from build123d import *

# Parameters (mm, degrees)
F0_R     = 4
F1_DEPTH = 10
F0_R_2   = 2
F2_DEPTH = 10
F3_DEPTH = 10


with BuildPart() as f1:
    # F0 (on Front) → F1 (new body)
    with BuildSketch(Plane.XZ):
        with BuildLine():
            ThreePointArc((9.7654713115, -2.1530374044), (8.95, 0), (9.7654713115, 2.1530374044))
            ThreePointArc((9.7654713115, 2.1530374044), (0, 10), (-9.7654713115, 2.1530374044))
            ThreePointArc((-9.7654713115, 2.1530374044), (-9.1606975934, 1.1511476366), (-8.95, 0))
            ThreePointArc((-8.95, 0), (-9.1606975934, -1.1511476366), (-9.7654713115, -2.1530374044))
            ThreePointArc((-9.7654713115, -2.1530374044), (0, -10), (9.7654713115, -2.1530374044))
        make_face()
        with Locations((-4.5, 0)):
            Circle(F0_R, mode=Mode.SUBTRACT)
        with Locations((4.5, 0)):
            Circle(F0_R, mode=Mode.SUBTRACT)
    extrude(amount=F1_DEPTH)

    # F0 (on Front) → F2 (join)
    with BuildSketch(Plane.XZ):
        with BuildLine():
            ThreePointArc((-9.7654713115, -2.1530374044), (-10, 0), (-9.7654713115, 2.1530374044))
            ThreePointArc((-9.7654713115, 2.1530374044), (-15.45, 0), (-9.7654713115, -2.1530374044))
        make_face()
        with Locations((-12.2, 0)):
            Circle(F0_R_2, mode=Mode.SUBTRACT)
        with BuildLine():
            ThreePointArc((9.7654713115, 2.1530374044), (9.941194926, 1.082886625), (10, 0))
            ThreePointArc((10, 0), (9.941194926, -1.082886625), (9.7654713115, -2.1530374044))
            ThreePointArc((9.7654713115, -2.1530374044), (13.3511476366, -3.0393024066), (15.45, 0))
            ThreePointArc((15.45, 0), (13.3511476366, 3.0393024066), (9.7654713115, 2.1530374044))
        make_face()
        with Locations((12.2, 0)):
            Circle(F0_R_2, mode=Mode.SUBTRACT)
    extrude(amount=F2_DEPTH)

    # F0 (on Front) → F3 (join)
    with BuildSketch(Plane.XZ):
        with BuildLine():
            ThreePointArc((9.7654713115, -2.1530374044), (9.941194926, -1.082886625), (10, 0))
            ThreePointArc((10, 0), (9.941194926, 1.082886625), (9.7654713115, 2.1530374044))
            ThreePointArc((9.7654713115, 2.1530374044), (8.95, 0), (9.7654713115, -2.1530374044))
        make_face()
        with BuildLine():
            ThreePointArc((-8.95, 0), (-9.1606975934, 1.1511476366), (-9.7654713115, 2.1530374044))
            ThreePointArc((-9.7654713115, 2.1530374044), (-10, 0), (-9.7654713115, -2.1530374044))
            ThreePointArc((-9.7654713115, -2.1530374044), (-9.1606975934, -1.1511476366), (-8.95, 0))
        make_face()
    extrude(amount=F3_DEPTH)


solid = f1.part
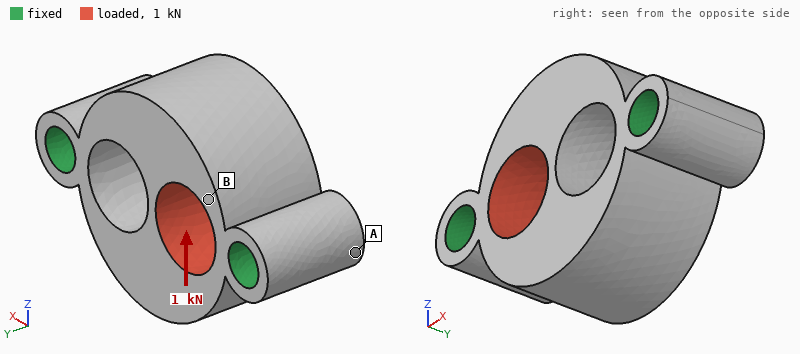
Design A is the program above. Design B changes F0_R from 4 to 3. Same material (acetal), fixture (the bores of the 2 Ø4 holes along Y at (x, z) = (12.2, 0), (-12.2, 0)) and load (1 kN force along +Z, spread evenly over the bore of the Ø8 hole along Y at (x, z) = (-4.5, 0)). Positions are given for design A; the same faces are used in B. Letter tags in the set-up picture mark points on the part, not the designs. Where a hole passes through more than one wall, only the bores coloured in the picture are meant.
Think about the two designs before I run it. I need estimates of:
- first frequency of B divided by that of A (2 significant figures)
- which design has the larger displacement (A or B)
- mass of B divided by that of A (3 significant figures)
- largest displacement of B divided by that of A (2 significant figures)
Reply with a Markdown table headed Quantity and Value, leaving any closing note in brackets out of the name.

| Quantity | Value |
|---|---|
| first frequency of B divided by that of A | 1.0 |
| which design has the larger displacement | A |
| mass of B divided by that of A | 1.18 |
| largest displacement of B divided by that of A | 0.80 |
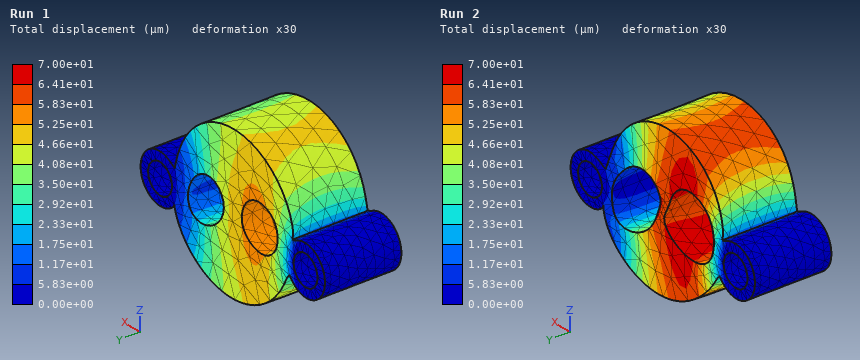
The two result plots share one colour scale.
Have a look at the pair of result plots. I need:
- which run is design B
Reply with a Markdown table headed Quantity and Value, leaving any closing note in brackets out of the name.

| Quantity | Value |
|---|---|
| which run is design B | Run 1 |
